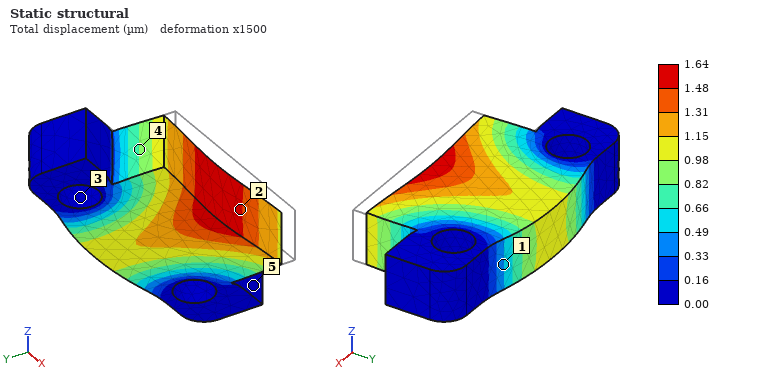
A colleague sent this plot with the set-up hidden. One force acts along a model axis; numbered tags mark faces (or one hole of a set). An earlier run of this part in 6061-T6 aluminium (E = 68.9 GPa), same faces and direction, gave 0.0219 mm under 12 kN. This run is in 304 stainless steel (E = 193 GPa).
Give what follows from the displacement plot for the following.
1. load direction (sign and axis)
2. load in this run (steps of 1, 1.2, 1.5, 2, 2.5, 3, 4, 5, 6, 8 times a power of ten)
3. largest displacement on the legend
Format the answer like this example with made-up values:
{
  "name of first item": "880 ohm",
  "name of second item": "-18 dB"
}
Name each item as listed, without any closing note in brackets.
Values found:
{
  "load direction": "+Y",
  "load in this run": "2.5 kN",
  "largest displacement on the legend": "1.64 µm"
}
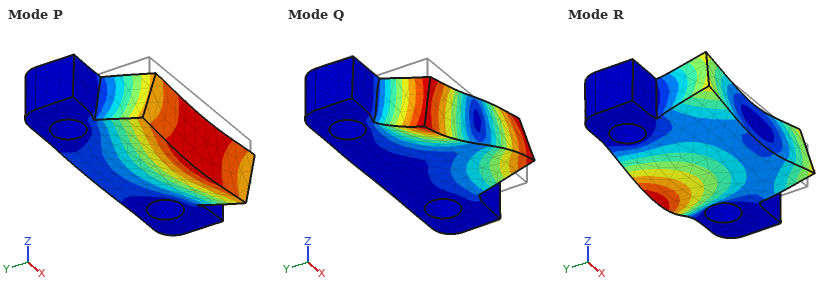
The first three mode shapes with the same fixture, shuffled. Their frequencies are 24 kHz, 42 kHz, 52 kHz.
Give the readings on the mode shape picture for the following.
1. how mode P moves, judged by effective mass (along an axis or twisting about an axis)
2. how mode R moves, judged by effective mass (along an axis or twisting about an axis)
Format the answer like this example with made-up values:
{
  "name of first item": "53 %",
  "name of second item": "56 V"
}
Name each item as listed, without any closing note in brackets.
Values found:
{
  "how mode P moves, judged by effective mass": "along Z",
  "how mode R moves, judged by effective mass": "along Z"
}
